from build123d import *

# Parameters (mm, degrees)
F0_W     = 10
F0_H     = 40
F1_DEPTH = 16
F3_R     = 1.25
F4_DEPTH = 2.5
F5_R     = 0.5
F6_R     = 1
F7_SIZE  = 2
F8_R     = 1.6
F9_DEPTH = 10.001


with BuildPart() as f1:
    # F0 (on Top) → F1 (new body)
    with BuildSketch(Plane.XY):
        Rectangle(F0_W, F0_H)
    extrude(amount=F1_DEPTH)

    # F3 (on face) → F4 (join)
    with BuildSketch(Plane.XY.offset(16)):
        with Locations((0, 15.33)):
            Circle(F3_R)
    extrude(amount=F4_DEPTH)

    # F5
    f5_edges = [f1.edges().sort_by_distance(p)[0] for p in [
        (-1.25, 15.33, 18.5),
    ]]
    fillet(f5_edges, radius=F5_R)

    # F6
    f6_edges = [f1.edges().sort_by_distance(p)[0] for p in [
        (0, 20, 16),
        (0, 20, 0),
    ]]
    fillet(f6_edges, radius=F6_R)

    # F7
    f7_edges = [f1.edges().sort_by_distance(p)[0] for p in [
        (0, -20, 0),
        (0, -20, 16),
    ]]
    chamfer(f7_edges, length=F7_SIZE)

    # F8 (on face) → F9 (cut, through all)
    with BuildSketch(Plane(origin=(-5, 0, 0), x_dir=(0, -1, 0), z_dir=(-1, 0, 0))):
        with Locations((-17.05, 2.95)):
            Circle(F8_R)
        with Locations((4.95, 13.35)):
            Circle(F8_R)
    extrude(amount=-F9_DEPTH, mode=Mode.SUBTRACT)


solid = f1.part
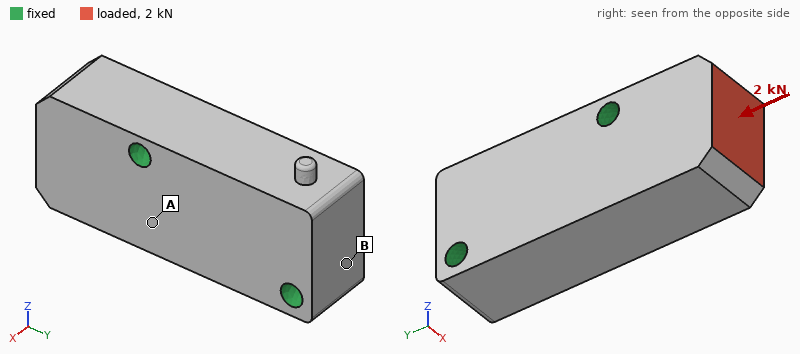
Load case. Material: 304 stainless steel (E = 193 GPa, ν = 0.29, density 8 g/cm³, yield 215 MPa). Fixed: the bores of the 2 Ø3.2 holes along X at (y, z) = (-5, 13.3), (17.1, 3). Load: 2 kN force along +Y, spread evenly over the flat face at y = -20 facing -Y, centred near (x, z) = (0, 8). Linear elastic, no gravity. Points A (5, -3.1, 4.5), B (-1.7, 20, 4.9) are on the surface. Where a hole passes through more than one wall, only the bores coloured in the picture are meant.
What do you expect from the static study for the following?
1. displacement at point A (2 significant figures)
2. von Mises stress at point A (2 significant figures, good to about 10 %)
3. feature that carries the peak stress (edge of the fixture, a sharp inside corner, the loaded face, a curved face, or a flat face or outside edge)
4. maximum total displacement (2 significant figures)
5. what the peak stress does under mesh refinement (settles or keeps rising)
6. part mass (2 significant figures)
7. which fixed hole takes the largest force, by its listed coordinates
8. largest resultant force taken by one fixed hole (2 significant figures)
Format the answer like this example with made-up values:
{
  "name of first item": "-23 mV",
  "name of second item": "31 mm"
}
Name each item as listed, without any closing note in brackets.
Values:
{
  "displacement at point A": "0.88 µm",
  "von Mises stress at point A": "11 MPa",
  "feature that carries the peak stress": "edge of the fixture",
  "maximum total displacement": "2.6 µm",
  "what the peak stress does under mesh refinement": "keeps rising",
  "part mass": "50 g",
  "which fixed hole takes the largest force, by its listed coordinates": "(-5, 13.3)",
  "largest resultant force taken by one fixed hole": "1.5 kN"
}
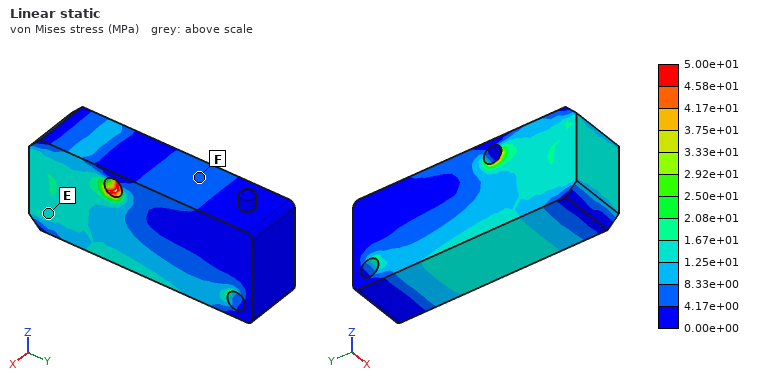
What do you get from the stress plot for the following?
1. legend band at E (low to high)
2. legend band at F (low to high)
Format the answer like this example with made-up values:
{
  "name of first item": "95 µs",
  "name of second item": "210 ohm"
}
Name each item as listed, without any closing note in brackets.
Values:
{
  "legend band at E": "1.25e+01 to 1.67e+01 MPa",
  "legend band at F": "4.17e+00 to 8.33e+00 MPa"
}
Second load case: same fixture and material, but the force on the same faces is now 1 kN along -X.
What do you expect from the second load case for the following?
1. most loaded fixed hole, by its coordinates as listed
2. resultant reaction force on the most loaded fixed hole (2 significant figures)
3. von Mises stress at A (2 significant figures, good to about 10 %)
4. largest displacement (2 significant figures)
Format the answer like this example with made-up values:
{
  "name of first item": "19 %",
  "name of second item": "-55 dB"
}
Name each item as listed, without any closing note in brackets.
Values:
{
  "most loaded fixed hole, by its coordinates as listed": "(-5, 13.3)",
  "resultant reaction force on the most loaded fixed hole": "1.2 kN",
  "von Mises stress at A": "25 MPa",
  "largest displacement": "9.7 µm"
}
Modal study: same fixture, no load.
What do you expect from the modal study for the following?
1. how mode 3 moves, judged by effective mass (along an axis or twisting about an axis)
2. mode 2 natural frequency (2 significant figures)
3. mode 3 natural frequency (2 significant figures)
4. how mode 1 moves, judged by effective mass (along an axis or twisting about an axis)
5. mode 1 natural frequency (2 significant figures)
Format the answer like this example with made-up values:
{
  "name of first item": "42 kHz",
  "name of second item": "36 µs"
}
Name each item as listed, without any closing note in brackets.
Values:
{
  "how mode 3 moves, judged by effective mass": "twisting about Y",
  "mode 2 natural frequency": "25 kHz",
  "mode 3 natural frequency": "32 kHz",
  "how mode 1 moves, judged by effective mass": "along X",
  "mode 1 natural frequency": "20 kHz"
}
